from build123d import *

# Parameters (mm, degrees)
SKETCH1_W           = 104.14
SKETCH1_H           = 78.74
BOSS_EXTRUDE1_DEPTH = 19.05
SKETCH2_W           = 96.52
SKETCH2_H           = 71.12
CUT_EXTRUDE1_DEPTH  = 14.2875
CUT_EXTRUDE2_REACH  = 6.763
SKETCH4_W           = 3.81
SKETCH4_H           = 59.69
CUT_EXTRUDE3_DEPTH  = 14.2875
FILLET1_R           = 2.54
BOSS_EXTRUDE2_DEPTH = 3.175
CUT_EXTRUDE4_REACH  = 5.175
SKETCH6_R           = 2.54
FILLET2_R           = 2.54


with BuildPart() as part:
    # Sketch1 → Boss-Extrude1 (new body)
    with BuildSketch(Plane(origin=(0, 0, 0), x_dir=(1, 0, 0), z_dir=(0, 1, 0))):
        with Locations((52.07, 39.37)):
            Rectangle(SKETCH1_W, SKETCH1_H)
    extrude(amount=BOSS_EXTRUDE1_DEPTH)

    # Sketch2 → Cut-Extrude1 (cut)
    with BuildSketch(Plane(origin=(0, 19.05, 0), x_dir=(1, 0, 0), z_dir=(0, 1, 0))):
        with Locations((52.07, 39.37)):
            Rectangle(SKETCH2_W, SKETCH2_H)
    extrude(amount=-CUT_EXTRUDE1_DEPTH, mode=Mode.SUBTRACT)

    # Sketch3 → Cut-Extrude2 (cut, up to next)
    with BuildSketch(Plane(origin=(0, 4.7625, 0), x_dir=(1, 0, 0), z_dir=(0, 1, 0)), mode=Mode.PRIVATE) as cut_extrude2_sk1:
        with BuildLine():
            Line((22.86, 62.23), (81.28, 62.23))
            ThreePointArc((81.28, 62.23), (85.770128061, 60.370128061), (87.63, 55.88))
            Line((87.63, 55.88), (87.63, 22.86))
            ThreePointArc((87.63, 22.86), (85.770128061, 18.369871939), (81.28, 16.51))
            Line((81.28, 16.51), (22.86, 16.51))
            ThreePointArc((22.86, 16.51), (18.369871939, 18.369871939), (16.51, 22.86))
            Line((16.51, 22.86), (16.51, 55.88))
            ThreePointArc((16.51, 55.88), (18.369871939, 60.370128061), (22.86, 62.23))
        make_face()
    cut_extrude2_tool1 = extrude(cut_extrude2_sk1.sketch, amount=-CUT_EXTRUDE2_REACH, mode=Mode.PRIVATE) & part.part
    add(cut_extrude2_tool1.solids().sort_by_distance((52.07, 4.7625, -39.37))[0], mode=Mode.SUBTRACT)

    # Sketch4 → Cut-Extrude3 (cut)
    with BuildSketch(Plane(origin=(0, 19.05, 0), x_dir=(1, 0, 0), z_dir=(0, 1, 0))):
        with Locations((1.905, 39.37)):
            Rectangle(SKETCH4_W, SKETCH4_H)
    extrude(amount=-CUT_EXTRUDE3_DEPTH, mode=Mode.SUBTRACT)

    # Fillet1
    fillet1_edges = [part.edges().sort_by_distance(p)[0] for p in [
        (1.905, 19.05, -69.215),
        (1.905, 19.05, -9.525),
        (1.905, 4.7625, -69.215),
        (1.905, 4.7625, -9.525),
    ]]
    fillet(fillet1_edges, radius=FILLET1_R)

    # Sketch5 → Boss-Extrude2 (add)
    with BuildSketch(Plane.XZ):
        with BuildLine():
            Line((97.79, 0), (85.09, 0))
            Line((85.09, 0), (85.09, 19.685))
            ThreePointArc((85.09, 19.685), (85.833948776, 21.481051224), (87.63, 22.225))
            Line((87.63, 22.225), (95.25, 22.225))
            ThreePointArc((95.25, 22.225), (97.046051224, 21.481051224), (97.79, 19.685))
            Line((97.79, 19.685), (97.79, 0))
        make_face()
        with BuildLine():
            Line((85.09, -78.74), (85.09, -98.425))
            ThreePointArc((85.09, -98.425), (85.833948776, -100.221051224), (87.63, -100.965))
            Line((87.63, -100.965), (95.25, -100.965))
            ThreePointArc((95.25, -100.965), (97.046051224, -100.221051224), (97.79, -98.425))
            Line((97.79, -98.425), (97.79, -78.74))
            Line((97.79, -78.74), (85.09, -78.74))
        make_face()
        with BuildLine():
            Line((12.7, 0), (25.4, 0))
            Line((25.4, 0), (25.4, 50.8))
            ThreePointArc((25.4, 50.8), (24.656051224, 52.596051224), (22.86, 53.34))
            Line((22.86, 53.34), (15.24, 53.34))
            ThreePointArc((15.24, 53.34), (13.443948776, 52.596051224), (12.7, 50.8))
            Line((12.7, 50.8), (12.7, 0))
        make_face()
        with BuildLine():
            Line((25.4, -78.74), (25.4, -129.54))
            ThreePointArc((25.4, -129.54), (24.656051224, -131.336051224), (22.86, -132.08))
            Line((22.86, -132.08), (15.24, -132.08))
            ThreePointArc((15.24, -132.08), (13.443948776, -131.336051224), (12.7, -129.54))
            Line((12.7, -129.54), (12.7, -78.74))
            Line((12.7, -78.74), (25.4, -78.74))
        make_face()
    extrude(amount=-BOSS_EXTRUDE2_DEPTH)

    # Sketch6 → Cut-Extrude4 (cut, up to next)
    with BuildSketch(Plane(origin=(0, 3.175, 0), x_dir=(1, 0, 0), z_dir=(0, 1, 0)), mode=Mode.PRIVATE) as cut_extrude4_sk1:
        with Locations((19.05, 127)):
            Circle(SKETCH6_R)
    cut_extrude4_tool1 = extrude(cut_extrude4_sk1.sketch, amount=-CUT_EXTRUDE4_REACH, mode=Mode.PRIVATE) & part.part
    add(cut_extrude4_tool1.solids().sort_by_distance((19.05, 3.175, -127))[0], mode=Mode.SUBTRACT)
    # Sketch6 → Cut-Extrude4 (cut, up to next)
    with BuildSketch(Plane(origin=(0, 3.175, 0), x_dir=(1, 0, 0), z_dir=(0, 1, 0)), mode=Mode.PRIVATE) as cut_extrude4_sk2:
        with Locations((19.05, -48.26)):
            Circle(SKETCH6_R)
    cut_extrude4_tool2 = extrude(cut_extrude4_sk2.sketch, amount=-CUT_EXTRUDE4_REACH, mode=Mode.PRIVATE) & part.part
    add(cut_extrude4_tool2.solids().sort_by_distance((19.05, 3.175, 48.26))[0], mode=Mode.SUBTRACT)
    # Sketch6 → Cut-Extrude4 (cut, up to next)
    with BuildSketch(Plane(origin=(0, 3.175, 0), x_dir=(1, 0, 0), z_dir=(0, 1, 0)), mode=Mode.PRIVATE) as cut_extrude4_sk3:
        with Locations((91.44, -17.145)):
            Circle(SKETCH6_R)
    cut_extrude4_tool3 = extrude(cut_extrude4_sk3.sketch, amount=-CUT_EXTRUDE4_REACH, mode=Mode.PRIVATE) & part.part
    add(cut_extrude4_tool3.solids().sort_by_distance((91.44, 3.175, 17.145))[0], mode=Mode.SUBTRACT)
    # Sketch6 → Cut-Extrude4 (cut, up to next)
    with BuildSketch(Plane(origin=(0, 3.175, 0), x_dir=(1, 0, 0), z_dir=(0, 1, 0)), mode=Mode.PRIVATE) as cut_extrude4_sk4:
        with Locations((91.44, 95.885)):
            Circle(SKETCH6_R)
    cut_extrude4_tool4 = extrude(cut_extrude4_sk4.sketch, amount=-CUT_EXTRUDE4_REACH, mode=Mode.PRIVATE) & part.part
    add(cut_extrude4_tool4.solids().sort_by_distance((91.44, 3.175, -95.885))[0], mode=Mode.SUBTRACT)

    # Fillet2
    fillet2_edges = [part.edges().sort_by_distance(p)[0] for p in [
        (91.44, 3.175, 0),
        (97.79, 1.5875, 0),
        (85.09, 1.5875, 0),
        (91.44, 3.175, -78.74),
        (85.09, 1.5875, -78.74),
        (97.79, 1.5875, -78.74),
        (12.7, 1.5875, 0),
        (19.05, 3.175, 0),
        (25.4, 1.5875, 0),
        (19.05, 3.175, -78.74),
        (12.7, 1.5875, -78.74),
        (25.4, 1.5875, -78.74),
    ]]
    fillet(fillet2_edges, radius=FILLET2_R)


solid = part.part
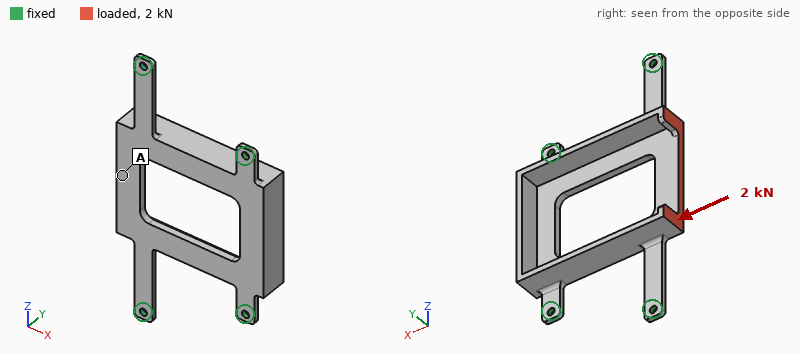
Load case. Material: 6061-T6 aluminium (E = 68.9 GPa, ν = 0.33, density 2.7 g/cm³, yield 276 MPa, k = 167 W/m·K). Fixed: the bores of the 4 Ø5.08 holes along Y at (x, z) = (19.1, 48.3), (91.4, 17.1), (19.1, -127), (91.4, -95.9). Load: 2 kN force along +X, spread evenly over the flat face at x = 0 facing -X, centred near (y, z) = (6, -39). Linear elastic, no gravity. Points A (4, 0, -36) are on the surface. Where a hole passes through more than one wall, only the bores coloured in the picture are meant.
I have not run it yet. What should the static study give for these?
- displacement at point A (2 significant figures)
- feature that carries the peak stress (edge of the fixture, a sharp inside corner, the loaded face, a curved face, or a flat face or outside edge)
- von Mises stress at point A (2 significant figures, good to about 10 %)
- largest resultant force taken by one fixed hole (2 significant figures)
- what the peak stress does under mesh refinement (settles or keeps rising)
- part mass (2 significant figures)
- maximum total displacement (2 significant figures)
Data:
0.32 mm
edge of the fixture
17 MPa
890 N
keeps rising
120 g
0.34 mm
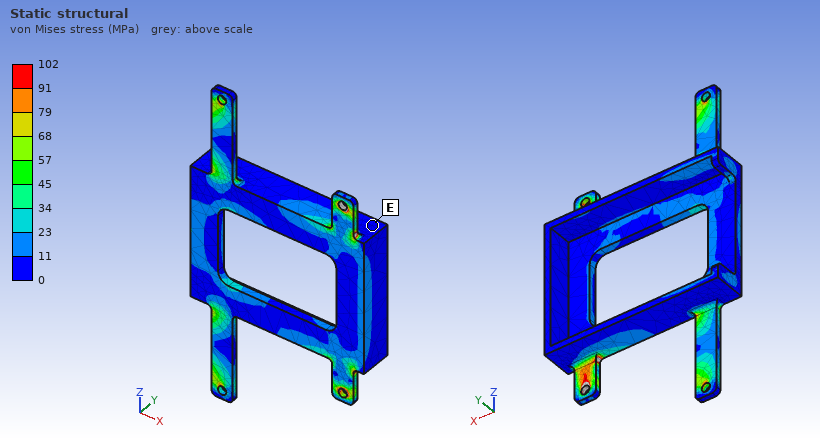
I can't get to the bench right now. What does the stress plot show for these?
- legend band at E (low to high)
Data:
0 to 11 MPa
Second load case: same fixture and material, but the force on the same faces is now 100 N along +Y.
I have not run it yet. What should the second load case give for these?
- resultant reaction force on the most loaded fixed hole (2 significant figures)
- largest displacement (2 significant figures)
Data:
88 N
0.37 mm
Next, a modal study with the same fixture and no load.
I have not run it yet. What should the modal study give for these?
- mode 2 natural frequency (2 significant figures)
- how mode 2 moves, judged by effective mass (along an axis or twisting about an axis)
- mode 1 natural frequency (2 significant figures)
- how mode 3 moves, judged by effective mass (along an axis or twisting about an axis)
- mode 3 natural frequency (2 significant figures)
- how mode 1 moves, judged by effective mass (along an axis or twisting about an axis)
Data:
1100 Hz
twisting about X
470 Hz
along Y
2000 Hz
along Y
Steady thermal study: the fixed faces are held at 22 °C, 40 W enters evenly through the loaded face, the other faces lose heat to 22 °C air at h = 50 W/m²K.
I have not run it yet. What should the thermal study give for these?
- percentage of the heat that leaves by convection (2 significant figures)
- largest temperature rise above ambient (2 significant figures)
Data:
60 %
47 K
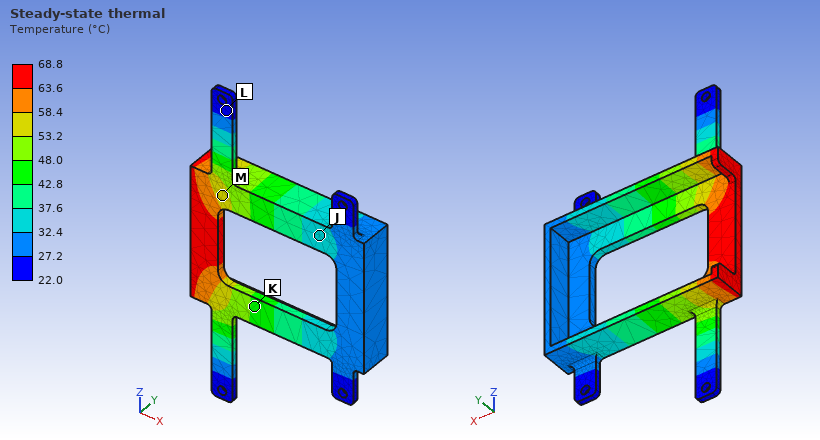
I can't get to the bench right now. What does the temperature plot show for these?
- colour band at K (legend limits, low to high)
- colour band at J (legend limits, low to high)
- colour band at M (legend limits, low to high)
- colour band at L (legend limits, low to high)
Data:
42.8 to 48.0 °C
32.4 to 37.6 °C
53.2 to 58.4 °C
22.0 to 27.2 °C
